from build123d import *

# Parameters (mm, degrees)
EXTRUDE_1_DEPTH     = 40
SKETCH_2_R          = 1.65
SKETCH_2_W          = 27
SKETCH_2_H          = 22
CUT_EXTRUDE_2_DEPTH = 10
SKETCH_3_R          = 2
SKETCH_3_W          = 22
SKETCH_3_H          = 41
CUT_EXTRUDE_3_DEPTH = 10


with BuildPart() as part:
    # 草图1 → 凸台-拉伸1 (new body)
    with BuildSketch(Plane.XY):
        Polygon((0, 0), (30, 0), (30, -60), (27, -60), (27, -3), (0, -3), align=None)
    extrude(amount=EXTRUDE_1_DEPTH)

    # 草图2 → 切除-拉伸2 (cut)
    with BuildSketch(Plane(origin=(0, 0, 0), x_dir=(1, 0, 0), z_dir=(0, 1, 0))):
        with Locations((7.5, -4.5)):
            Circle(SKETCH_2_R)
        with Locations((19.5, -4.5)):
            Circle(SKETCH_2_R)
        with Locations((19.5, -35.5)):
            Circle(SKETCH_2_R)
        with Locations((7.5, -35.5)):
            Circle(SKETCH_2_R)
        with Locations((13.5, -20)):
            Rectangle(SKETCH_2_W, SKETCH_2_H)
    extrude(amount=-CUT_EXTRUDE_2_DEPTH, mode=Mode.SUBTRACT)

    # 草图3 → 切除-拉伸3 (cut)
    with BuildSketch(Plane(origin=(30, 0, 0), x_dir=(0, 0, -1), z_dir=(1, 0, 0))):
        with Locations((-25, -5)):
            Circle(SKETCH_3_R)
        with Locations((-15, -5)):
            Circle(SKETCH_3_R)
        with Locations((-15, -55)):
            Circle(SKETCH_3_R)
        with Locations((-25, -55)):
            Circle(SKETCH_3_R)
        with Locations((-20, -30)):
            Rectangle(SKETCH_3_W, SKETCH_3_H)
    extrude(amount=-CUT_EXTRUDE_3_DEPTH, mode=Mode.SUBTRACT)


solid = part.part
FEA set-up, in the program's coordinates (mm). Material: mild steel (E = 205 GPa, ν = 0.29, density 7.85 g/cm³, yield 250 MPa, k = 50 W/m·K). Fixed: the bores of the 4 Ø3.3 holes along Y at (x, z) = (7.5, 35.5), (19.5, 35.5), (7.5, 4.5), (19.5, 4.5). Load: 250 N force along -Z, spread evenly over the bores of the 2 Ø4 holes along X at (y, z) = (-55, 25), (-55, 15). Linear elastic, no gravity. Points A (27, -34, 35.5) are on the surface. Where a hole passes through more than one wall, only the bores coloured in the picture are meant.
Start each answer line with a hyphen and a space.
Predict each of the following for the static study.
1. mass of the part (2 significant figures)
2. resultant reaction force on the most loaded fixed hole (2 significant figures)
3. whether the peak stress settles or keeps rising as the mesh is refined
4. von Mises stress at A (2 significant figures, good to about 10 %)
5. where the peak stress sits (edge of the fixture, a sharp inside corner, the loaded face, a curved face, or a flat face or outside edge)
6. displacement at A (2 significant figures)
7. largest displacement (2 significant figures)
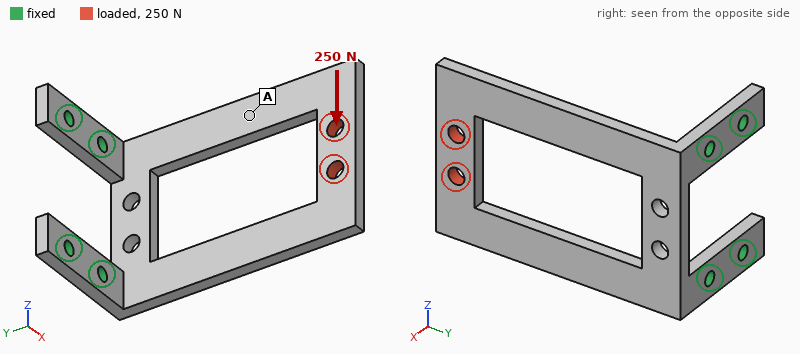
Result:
- 45 g
- 420 N
- keeps rising
- 25 MPa
- edge of the fixture
- 0.066 mm
- 0.11 mm
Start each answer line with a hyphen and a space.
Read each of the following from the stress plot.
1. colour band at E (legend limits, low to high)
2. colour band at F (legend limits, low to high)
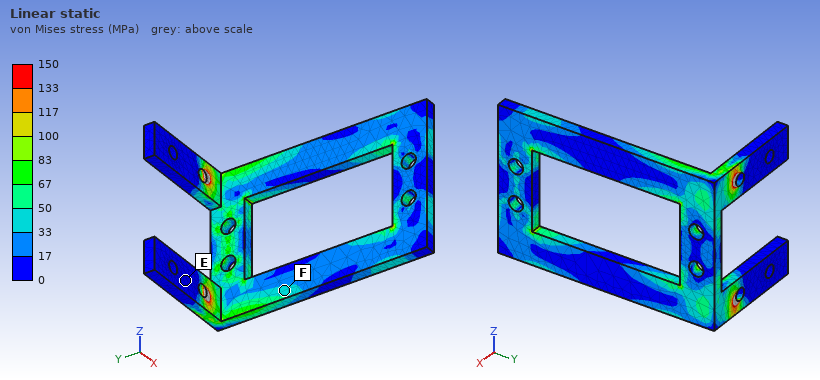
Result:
- 0 to 17 MPa
- 33 to 50 MPa
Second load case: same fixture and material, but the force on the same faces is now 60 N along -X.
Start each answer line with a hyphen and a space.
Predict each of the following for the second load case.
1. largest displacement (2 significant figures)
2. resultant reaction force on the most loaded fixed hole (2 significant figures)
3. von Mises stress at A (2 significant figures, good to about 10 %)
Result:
- 0.56 mm
- 30 N
- 47 MPa
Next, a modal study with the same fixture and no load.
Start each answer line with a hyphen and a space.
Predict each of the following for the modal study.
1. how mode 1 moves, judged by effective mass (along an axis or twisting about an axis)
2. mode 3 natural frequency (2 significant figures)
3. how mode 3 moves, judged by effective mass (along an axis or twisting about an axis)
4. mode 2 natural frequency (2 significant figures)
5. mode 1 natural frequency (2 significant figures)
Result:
- along X
- 2200 Hz
- along Z
- 1600 Hz
- 490 Hz
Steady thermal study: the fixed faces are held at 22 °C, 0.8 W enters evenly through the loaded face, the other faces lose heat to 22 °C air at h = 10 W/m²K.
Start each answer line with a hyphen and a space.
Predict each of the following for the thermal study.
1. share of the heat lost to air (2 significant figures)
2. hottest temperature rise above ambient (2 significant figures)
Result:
- 36 %
- 15 K
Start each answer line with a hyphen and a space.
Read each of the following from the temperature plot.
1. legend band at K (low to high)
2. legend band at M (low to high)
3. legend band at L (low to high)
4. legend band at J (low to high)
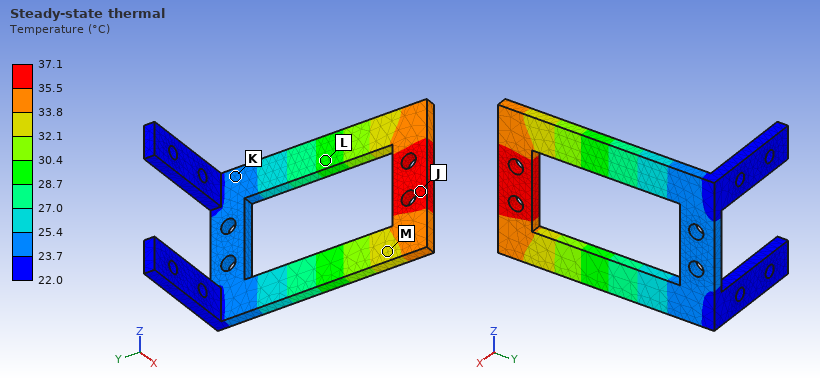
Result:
- 23.7 to 25.4 °C
- 32.1 to 33.8 °C
- 28.7 to 30.4 °C
- 35.5 to 37.1 °C
